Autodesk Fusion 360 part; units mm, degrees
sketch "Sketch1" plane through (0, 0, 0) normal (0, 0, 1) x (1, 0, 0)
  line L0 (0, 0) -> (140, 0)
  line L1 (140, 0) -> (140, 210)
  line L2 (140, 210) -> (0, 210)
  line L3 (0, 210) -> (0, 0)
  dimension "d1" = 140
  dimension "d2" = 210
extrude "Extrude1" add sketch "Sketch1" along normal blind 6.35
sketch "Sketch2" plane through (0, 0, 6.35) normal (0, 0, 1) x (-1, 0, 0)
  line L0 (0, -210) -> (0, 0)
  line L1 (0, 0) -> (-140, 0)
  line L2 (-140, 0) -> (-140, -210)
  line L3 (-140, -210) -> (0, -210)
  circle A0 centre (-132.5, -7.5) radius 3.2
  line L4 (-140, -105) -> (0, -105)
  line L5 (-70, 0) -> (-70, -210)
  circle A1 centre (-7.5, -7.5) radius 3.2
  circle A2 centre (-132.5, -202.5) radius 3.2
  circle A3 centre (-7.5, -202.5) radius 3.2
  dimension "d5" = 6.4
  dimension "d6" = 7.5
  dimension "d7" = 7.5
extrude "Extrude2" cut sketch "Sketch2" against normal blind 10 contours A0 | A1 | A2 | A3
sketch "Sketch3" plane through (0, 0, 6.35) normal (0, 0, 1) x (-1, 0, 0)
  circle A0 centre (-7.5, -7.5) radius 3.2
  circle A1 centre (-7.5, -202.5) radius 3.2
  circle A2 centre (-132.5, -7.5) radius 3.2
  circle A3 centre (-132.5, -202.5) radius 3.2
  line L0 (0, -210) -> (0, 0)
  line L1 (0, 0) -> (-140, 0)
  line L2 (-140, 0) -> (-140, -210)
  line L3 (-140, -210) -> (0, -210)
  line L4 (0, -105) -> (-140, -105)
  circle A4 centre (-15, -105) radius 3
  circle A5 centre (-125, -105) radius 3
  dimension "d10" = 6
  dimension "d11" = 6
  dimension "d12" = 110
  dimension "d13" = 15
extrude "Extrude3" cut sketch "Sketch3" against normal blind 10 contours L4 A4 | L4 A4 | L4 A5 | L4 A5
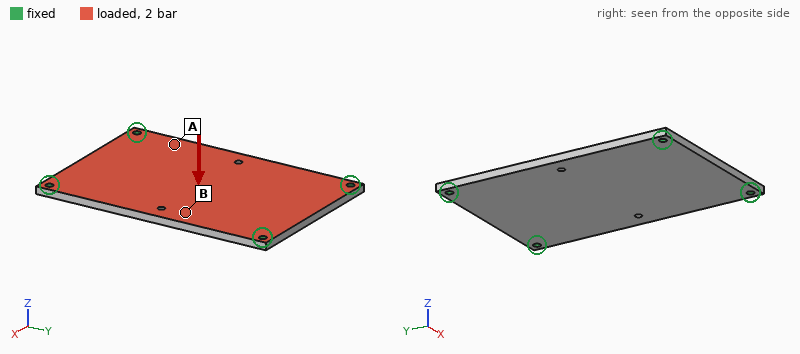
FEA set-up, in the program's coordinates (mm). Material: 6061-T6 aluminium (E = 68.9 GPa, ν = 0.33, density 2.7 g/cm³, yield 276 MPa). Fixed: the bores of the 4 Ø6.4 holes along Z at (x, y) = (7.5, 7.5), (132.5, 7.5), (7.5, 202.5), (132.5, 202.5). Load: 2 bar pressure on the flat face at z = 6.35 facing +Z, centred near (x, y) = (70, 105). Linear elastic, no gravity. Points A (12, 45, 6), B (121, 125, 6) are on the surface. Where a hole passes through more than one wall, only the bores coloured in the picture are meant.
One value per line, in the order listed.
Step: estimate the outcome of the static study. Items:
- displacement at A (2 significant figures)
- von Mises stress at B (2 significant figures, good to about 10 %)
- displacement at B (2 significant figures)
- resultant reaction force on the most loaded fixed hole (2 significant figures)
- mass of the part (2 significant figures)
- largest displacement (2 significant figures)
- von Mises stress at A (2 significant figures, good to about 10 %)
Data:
0.36 mm
55 MPa
0.78 mm
1.5 kN
500 g
0.88 mm
20 MPa
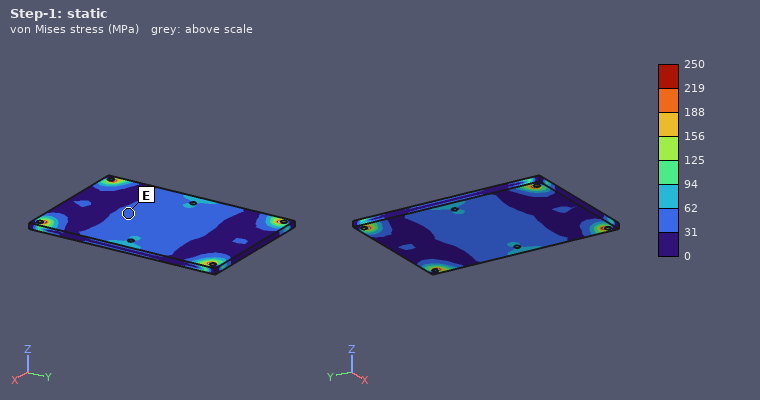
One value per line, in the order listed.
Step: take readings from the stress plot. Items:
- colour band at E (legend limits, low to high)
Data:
31 to 62 MPa
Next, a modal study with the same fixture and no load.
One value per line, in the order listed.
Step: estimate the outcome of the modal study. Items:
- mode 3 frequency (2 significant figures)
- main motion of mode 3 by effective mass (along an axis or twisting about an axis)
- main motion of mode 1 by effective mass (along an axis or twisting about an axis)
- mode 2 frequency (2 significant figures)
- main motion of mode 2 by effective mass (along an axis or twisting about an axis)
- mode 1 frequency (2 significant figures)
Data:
1700 Hz
twisting about X
along Z
1100 Hz
twisting about Y
670 Hz
